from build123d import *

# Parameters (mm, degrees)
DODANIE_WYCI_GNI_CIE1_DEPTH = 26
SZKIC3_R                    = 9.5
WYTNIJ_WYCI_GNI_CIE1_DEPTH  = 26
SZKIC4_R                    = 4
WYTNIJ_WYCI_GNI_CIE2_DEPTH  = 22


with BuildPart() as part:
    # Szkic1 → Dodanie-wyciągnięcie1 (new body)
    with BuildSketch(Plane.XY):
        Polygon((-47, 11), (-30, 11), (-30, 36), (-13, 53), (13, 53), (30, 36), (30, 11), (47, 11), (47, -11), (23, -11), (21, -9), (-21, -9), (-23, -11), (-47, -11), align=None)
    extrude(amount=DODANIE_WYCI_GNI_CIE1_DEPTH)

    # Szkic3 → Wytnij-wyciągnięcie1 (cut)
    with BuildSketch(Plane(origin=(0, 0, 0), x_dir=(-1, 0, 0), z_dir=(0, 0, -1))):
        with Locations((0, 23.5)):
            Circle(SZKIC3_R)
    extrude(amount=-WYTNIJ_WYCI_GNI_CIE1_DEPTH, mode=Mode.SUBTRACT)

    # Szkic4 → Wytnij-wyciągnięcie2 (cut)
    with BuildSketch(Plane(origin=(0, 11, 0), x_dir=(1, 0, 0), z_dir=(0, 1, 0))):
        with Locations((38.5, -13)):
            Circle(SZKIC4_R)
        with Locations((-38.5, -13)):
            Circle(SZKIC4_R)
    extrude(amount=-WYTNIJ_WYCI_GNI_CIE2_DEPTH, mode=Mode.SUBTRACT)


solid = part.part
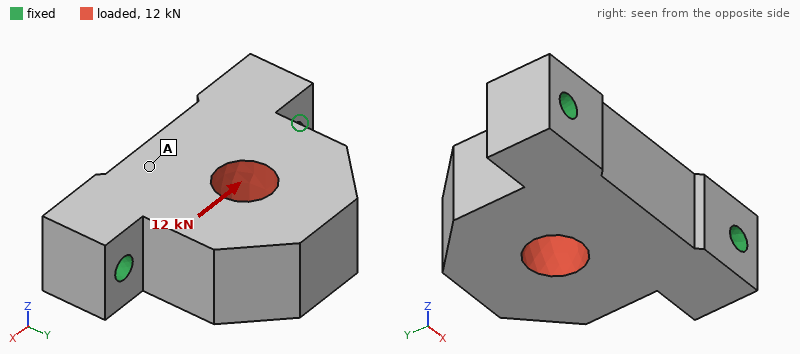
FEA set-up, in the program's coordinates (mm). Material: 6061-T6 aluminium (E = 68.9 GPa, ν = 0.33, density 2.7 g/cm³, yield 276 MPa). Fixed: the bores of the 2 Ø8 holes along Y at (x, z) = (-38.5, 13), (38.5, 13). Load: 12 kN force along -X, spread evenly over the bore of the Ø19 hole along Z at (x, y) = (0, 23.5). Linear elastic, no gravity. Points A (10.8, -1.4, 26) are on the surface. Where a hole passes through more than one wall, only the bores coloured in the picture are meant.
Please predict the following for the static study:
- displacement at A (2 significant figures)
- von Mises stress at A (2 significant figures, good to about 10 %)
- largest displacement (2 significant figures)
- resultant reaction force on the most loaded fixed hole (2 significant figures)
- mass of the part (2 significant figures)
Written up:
2.8 µm
4.6 MPa
18 µm
7.1 kN
270 g
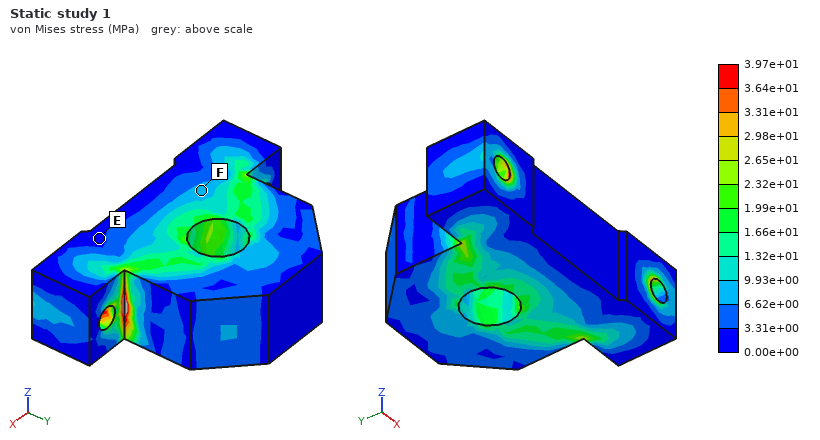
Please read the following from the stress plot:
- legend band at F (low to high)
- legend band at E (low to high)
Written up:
6.62e+00 to 9.93e+00 MPa
0.00e+00 to 3.31e+00 MPa
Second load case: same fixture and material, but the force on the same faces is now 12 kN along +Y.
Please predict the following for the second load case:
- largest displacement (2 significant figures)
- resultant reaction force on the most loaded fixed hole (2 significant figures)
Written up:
14 µm
6.5 kN
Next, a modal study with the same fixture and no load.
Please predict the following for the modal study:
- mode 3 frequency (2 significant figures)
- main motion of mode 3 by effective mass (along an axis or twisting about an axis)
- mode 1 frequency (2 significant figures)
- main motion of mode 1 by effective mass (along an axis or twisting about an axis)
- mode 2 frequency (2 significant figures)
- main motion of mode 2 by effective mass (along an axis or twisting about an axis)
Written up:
11 kHz
along Y
4100 Hz
along Z
10 kHz
along X
